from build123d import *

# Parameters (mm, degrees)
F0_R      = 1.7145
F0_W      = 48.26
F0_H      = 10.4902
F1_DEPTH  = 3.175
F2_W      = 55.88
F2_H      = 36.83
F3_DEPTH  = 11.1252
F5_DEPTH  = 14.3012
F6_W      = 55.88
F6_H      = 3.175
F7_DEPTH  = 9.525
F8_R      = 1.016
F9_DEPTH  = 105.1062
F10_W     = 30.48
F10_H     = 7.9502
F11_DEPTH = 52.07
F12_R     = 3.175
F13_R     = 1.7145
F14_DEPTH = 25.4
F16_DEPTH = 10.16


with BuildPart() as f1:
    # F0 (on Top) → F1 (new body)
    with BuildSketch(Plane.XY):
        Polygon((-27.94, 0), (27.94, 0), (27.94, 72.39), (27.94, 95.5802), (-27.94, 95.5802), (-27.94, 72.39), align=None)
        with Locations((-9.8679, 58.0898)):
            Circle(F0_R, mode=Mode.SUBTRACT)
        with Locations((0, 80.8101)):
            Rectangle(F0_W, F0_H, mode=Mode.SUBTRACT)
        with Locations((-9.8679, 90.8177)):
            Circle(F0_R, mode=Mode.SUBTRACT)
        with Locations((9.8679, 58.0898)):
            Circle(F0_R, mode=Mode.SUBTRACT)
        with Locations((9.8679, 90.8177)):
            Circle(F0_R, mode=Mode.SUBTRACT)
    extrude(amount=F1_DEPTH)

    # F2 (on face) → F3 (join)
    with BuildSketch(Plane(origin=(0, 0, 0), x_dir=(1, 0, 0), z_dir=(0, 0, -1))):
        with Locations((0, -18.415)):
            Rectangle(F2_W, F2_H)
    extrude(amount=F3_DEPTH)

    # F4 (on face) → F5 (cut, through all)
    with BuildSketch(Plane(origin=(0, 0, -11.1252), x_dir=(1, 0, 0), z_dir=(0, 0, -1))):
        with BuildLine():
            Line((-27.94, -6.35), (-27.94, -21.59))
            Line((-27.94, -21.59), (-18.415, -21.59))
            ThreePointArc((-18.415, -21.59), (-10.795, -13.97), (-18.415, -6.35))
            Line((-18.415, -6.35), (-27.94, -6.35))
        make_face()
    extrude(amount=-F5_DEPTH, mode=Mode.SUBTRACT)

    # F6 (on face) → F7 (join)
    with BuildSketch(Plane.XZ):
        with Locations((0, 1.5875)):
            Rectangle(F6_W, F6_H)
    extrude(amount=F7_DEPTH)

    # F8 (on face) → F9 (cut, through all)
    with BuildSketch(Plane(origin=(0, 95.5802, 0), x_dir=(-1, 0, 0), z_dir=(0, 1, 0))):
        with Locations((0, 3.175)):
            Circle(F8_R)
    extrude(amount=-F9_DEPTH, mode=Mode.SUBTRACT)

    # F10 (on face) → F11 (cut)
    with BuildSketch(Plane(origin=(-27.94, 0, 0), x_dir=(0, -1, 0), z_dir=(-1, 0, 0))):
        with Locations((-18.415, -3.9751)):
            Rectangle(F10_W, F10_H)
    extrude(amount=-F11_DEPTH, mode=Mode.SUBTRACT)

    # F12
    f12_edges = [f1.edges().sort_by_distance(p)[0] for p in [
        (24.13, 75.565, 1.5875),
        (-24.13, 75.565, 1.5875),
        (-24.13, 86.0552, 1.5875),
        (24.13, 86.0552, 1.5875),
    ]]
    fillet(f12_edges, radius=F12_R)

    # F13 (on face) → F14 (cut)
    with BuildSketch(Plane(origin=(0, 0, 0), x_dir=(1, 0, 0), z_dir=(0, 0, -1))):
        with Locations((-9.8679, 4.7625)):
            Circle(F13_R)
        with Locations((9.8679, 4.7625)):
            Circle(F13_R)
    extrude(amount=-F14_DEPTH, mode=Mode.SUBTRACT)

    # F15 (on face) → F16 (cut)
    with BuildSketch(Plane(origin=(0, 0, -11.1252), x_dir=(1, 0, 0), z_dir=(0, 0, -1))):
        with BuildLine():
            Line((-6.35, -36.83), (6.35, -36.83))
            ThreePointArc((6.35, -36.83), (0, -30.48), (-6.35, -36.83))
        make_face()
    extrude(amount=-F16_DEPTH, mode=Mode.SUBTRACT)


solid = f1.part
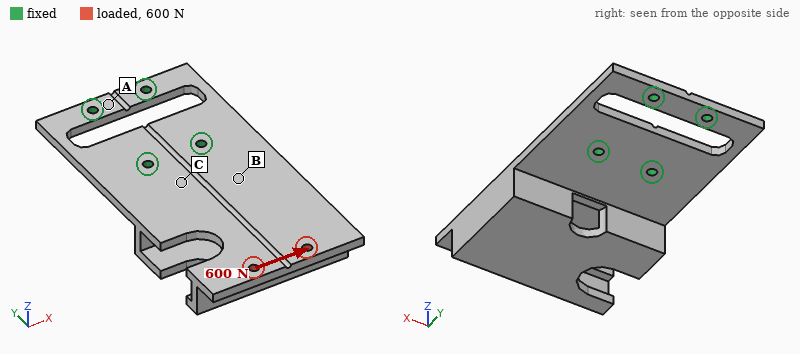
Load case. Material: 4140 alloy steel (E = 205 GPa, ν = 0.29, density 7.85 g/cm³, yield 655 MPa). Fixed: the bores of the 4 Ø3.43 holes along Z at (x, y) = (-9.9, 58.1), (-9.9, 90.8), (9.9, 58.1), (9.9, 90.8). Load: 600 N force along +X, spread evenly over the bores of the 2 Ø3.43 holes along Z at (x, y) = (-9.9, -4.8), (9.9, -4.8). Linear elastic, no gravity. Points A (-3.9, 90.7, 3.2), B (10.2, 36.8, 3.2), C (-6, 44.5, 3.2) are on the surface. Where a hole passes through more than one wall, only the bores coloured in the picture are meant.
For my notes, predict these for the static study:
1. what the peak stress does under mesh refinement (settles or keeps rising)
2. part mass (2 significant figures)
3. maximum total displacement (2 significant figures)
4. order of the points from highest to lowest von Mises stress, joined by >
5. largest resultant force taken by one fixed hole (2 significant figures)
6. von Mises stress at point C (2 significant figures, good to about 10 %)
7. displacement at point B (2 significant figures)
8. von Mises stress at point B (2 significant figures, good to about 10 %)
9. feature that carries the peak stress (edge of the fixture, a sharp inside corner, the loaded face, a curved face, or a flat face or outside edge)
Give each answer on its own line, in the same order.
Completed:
keeps rising
200 g
23 µm
C > B > A
1.4 kN
19 MPa
5.1 µm
11 MPa
edge of the fixture
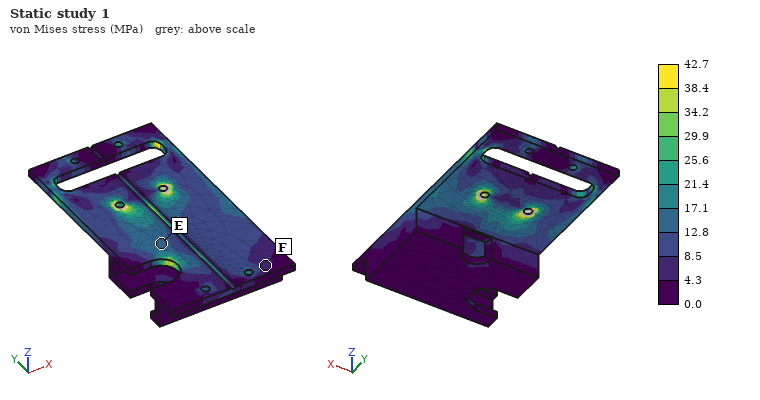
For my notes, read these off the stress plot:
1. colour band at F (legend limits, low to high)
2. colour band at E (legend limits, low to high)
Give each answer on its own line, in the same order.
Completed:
4.3 to 8.5 MPa
12.8 to 17.1 MPa
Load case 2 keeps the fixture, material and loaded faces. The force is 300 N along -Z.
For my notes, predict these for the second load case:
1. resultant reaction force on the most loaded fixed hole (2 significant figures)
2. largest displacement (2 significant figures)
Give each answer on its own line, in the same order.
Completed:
200 N
0.75 mm
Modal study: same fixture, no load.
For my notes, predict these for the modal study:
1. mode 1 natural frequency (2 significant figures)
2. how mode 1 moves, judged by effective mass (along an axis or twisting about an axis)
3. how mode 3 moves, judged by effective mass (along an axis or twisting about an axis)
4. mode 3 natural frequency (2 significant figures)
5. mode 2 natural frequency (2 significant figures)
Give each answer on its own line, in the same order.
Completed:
440 Hz
along Z
along X
3600 Hz
1700 Hz
